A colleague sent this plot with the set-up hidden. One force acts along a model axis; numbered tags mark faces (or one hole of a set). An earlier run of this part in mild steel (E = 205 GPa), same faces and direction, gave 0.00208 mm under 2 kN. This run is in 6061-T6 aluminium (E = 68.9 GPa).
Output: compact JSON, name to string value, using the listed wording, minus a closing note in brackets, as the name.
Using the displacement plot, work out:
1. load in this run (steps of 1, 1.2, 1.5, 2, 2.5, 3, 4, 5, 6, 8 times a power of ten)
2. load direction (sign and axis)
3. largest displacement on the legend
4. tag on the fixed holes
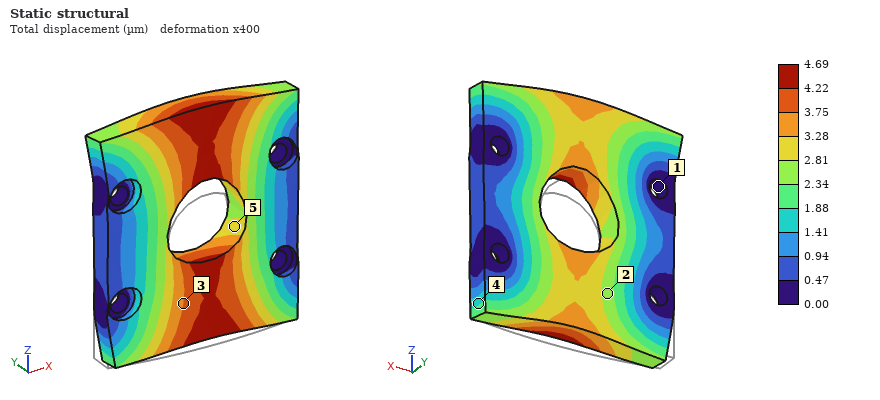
{"load in this run": "1.5 kN", "load direction": "+Z", "largest displacement on the legend": "4.69 µm", "tag on the fixed holes": "1"}
